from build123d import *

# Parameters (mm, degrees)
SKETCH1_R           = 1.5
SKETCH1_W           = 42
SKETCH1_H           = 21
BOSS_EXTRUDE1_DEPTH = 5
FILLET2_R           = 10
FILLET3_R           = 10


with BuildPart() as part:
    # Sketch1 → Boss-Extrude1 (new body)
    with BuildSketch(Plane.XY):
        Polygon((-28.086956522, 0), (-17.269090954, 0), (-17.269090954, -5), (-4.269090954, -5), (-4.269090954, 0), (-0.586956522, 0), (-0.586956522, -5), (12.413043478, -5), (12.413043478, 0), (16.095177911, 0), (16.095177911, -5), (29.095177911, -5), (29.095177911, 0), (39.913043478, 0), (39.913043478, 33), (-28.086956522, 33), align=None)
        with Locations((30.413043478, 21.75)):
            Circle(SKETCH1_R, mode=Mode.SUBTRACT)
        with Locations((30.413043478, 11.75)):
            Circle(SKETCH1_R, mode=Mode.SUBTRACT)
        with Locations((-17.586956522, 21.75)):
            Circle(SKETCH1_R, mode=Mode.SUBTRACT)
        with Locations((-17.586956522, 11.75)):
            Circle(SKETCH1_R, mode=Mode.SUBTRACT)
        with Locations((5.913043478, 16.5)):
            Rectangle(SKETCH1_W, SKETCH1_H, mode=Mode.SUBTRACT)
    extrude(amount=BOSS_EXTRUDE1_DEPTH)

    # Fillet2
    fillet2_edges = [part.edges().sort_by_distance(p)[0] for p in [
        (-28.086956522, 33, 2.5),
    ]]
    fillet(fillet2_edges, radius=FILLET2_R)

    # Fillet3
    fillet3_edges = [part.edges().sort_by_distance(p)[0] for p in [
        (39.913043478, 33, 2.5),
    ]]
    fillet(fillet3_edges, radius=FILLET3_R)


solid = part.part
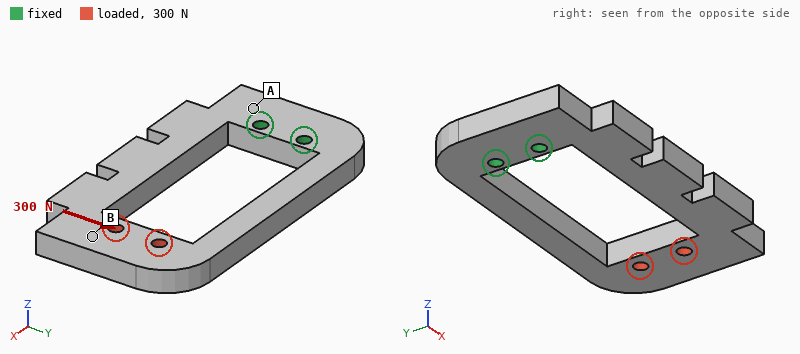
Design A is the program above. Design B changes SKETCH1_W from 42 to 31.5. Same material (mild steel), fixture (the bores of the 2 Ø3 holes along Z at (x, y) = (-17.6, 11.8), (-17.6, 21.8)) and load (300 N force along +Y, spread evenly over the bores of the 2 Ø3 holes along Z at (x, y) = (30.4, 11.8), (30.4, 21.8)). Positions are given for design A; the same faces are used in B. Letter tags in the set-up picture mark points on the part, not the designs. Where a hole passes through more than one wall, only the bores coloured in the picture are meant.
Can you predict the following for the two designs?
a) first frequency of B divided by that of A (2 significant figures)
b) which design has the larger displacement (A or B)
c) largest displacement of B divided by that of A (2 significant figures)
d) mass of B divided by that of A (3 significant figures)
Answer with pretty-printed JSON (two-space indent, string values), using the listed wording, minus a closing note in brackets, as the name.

{
  "first frequency of B divided by that of A": "1.1",
  "which design has the larger displacement": "A",
  "largest displacement of B divided by that of A": "0.52",
  "mass of B divided by that of A": "1.15"
}
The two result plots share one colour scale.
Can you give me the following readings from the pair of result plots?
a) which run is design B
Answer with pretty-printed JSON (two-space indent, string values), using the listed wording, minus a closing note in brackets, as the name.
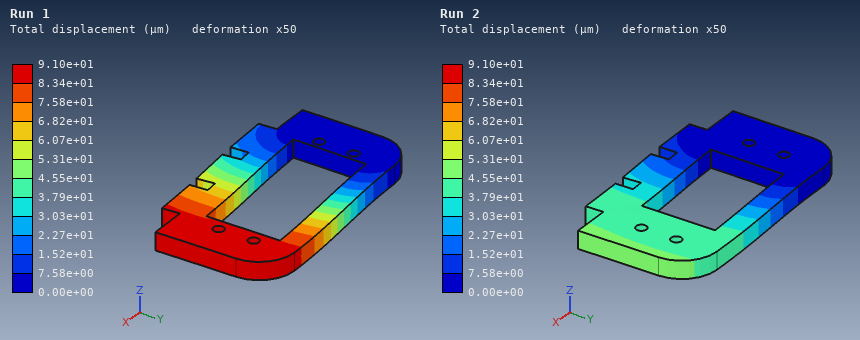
{
  "which run is design B": "Run 2"
}
